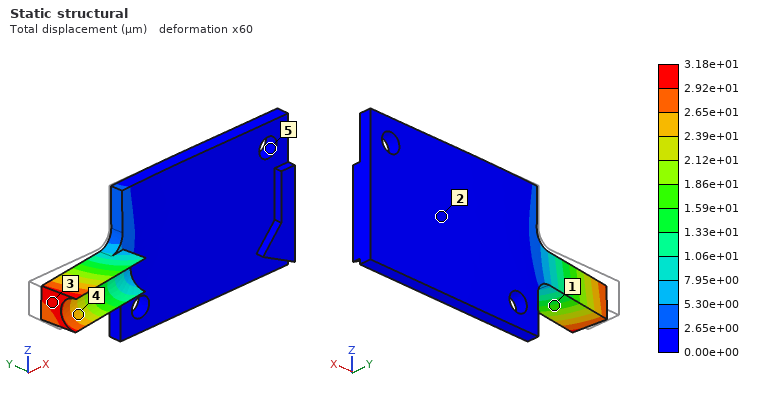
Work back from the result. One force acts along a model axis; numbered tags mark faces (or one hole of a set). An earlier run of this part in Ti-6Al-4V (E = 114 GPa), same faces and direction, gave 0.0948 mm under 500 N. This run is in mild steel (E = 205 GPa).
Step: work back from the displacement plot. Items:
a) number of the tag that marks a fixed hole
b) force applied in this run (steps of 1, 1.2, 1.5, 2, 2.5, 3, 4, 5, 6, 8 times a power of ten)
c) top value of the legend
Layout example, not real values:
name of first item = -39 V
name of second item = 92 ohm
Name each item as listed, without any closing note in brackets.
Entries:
number of the tag that marks a fixed hole = 5
force applied in this run = 300 N
top value of the legend = 3.18e+01 µm
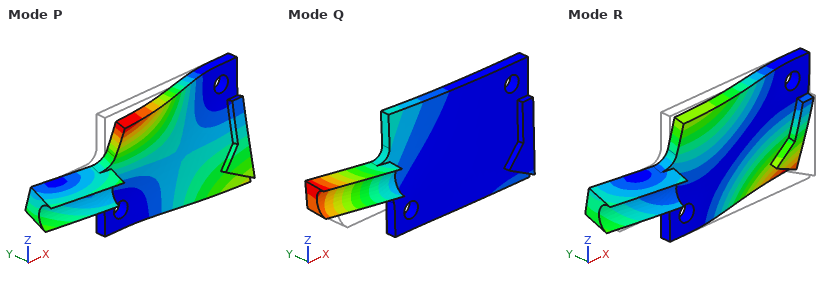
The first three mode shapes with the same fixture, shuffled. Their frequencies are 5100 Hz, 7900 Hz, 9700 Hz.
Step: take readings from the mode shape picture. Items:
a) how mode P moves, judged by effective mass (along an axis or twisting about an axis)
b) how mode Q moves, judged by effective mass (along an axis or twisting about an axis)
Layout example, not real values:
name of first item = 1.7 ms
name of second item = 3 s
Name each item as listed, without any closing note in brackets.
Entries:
how mode P moves, judged by effective mass = along Y
how mode Q moves, judged by effective mass = along Y
